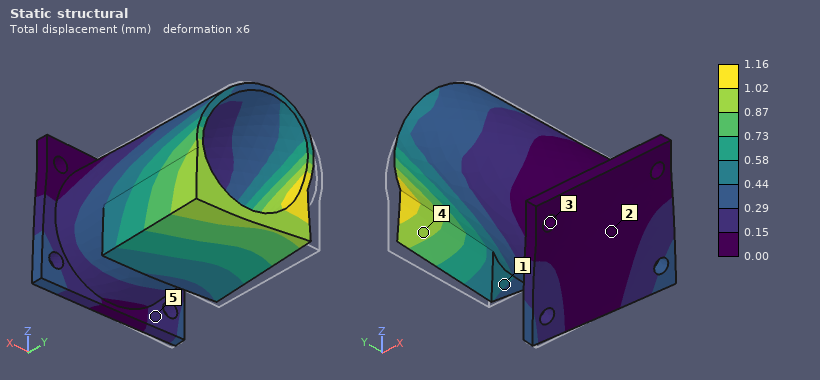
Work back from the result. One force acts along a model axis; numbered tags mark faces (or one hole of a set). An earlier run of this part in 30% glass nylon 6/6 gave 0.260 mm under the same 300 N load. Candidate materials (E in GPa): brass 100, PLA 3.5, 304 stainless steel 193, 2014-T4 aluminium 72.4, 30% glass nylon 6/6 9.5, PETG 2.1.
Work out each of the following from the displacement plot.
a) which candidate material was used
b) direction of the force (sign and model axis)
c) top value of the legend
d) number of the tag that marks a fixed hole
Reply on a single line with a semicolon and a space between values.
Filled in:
PETG; +X; 1.16 mm; 3
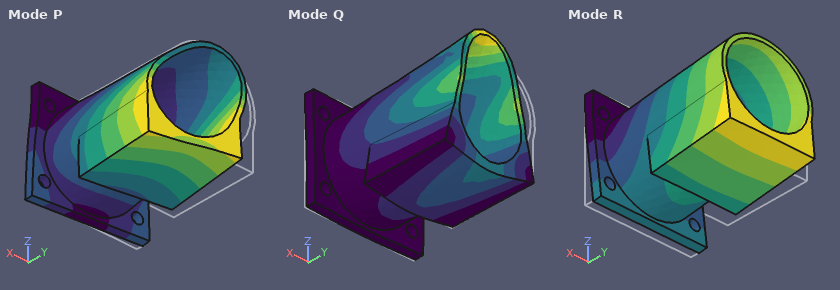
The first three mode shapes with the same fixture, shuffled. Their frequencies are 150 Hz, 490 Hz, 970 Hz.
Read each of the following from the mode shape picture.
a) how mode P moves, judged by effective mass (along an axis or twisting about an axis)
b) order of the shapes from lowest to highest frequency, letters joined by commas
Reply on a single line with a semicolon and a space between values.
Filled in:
along X; R, P, Q
